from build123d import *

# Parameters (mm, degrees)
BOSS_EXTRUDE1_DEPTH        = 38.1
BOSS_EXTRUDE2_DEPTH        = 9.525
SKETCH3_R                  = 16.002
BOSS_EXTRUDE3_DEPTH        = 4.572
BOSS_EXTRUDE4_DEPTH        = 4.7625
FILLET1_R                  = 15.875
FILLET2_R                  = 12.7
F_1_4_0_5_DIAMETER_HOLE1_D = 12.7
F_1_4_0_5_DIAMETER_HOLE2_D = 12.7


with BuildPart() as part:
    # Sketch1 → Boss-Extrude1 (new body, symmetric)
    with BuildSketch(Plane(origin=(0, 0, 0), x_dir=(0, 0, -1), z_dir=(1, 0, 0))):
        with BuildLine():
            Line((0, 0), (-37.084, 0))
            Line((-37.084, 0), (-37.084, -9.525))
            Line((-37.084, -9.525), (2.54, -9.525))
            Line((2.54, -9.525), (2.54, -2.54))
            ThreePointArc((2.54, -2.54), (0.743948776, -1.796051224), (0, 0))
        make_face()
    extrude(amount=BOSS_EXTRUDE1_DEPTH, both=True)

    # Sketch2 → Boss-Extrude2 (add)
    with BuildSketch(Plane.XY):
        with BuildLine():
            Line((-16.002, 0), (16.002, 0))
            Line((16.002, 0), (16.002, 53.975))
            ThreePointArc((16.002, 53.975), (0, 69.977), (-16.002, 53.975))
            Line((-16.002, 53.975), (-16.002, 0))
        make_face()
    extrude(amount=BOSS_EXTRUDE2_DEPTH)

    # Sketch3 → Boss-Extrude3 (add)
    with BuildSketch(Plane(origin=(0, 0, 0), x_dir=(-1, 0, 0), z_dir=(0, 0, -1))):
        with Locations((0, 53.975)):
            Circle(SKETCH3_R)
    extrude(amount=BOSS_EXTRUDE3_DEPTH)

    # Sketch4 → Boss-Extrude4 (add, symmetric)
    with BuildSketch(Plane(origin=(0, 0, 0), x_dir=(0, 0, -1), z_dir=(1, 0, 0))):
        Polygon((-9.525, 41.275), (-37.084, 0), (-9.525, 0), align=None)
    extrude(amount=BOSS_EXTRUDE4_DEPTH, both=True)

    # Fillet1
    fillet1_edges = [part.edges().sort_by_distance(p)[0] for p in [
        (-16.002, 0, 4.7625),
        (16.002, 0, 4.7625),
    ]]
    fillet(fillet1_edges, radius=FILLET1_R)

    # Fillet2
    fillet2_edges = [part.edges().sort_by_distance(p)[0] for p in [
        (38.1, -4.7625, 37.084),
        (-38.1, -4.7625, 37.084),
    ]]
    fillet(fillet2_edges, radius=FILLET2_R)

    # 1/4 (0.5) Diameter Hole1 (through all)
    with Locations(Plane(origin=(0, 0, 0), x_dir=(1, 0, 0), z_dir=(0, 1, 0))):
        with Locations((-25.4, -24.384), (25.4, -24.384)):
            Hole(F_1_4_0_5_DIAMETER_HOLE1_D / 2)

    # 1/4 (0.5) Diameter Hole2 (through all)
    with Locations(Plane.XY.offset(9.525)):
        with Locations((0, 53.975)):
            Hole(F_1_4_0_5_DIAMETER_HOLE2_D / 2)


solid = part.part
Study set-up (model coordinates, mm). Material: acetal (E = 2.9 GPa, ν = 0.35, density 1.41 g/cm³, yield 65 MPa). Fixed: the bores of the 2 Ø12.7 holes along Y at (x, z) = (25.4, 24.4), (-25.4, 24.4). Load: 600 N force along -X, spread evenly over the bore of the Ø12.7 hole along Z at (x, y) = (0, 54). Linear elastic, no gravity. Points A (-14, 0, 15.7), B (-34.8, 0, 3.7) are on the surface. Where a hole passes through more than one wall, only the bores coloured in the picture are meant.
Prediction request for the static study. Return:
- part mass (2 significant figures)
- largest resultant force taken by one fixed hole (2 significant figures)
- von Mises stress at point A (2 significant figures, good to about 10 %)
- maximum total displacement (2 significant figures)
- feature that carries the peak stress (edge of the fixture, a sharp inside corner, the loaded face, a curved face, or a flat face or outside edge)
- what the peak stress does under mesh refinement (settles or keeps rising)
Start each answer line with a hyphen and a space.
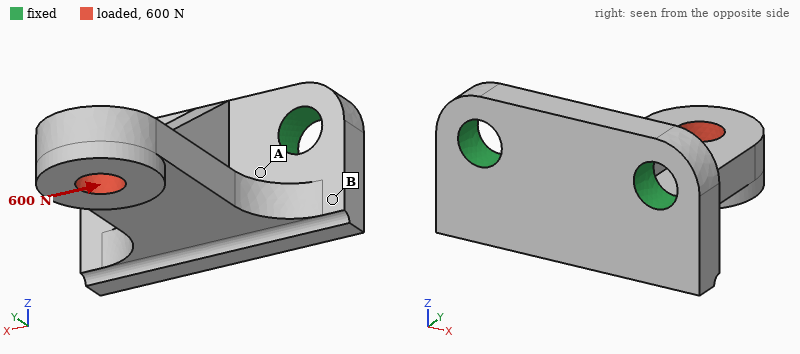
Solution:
- 76 g
- 860 N
- 6.1 MPa
- 1.1 mm
- edge of the fixture
- keeps rising
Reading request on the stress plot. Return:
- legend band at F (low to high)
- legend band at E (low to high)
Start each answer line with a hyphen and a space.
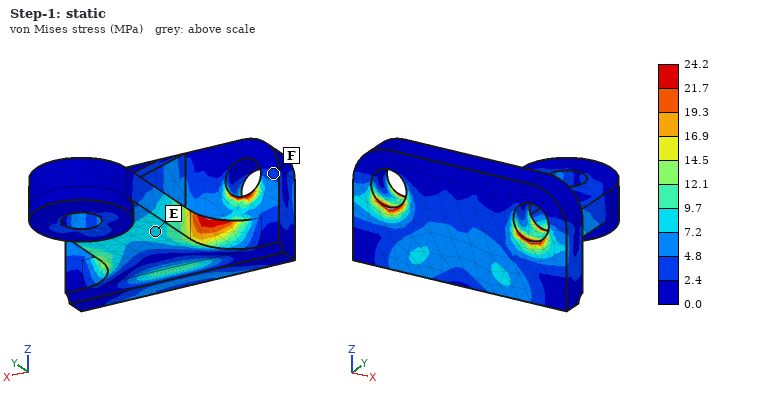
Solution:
- 2.4 to 4.8 MPa
- 7.2 to 9.7 MPa
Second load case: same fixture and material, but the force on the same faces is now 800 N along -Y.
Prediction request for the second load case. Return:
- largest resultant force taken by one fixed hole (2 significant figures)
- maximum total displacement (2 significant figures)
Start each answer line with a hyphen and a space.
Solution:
- 410 N
- 0.80 mm
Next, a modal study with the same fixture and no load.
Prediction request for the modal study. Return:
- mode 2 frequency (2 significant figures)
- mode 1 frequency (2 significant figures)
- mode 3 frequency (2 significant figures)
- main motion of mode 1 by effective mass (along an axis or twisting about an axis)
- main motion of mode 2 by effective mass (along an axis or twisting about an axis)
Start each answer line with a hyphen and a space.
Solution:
- 1000 Hz
- 650 Hz
- 2100 Hz
- along Z
- along X
